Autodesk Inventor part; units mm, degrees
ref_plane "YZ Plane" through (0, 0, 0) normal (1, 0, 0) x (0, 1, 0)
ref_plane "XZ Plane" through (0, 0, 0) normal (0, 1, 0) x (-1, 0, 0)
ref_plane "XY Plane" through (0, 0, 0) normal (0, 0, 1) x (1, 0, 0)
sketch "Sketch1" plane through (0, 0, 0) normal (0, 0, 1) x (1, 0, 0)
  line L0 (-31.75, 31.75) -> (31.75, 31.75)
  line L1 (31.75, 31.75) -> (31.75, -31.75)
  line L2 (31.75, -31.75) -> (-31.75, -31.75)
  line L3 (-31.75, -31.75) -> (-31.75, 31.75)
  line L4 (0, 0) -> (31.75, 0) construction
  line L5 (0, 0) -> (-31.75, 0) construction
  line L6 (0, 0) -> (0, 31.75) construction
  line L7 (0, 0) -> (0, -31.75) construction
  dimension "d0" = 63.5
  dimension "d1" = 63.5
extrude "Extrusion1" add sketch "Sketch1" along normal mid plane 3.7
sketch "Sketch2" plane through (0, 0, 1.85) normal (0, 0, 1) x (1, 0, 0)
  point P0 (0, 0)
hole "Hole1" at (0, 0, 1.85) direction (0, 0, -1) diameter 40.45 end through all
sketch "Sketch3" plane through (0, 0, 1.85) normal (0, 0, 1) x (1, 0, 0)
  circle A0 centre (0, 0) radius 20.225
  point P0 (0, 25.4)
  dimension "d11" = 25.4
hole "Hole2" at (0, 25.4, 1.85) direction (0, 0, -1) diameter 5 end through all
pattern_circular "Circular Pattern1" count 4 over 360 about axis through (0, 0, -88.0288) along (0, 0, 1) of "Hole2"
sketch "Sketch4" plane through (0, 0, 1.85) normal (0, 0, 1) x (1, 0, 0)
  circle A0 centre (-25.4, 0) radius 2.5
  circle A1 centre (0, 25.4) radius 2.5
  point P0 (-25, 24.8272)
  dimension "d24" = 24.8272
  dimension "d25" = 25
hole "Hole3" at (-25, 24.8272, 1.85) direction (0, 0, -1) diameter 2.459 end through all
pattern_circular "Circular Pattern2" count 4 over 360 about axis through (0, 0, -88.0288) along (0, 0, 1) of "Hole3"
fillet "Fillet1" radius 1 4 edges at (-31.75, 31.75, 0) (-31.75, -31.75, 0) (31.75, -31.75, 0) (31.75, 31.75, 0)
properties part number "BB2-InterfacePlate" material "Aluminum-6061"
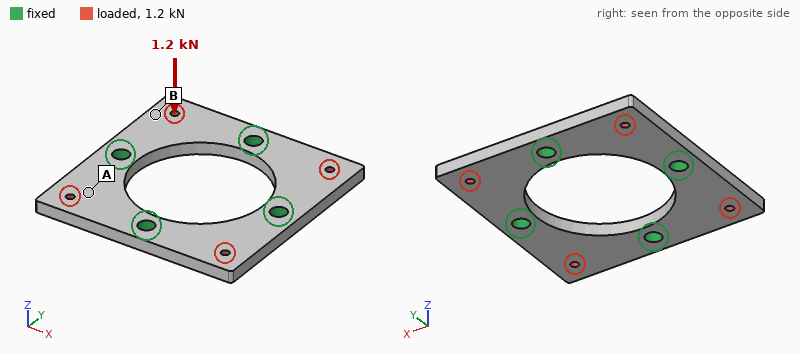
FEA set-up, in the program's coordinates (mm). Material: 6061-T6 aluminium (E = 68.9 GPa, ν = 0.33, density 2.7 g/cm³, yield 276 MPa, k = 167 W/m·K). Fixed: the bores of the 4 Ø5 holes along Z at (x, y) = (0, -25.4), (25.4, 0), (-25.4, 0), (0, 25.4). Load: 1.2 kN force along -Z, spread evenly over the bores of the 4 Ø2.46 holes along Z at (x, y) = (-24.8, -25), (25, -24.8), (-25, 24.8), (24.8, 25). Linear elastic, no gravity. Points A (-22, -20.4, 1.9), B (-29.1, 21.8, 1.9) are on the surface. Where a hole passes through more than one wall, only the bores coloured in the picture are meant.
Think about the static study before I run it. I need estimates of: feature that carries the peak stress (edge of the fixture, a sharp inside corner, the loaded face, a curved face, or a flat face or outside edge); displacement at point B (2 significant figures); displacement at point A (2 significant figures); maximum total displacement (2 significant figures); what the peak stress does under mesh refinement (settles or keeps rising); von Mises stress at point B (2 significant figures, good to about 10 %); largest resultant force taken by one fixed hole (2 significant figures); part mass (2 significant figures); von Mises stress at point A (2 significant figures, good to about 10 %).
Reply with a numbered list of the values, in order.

1. edge of the fixture
2. 0.098 mm
3. 0.062 mm
4. 0.16 mm
5. keeps rising
6. 28 MPa
7. 300 N
8. 26 g
9. 42 MPa
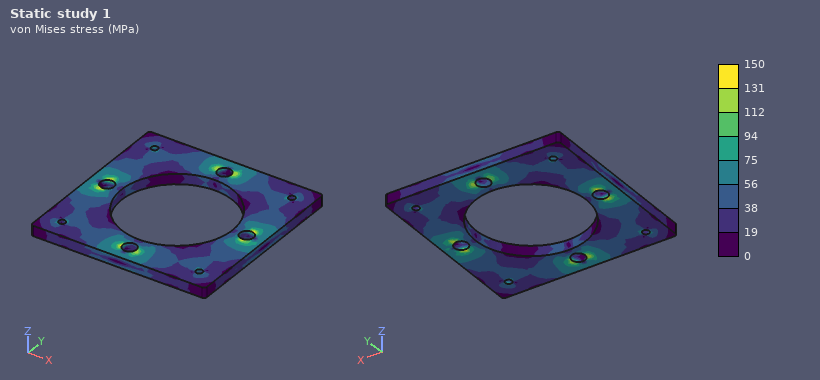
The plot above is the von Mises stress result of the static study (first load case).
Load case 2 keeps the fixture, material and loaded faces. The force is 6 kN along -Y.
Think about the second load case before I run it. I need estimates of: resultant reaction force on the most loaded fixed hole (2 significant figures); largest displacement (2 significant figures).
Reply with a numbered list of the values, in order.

1. 2.7 kN
2. 13 µm
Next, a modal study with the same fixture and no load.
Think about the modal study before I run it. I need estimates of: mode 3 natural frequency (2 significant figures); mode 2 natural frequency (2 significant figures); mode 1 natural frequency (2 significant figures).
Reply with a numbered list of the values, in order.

1. 5700 Hz
2. 5700 Hz
3. 5600 Hz
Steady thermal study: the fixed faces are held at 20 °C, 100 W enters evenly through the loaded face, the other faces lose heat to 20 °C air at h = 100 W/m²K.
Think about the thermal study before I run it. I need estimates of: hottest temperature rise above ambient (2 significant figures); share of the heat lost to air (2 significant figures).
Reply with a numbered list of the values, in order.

1. 42 K
2. 12 %
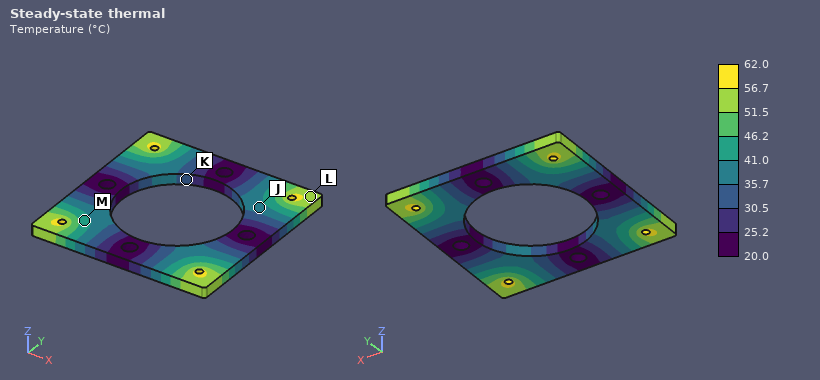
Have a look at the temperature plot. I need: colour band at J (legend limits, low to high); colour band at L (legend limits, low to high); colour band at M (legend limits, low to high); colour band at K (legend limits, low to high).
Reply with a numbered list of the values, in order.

1. 35.7 to 41.0 °C
2. 51.5 to 56.7 °C
3. 41.0 to 46.2 °C
4. 30.5 to 35.7 °C
